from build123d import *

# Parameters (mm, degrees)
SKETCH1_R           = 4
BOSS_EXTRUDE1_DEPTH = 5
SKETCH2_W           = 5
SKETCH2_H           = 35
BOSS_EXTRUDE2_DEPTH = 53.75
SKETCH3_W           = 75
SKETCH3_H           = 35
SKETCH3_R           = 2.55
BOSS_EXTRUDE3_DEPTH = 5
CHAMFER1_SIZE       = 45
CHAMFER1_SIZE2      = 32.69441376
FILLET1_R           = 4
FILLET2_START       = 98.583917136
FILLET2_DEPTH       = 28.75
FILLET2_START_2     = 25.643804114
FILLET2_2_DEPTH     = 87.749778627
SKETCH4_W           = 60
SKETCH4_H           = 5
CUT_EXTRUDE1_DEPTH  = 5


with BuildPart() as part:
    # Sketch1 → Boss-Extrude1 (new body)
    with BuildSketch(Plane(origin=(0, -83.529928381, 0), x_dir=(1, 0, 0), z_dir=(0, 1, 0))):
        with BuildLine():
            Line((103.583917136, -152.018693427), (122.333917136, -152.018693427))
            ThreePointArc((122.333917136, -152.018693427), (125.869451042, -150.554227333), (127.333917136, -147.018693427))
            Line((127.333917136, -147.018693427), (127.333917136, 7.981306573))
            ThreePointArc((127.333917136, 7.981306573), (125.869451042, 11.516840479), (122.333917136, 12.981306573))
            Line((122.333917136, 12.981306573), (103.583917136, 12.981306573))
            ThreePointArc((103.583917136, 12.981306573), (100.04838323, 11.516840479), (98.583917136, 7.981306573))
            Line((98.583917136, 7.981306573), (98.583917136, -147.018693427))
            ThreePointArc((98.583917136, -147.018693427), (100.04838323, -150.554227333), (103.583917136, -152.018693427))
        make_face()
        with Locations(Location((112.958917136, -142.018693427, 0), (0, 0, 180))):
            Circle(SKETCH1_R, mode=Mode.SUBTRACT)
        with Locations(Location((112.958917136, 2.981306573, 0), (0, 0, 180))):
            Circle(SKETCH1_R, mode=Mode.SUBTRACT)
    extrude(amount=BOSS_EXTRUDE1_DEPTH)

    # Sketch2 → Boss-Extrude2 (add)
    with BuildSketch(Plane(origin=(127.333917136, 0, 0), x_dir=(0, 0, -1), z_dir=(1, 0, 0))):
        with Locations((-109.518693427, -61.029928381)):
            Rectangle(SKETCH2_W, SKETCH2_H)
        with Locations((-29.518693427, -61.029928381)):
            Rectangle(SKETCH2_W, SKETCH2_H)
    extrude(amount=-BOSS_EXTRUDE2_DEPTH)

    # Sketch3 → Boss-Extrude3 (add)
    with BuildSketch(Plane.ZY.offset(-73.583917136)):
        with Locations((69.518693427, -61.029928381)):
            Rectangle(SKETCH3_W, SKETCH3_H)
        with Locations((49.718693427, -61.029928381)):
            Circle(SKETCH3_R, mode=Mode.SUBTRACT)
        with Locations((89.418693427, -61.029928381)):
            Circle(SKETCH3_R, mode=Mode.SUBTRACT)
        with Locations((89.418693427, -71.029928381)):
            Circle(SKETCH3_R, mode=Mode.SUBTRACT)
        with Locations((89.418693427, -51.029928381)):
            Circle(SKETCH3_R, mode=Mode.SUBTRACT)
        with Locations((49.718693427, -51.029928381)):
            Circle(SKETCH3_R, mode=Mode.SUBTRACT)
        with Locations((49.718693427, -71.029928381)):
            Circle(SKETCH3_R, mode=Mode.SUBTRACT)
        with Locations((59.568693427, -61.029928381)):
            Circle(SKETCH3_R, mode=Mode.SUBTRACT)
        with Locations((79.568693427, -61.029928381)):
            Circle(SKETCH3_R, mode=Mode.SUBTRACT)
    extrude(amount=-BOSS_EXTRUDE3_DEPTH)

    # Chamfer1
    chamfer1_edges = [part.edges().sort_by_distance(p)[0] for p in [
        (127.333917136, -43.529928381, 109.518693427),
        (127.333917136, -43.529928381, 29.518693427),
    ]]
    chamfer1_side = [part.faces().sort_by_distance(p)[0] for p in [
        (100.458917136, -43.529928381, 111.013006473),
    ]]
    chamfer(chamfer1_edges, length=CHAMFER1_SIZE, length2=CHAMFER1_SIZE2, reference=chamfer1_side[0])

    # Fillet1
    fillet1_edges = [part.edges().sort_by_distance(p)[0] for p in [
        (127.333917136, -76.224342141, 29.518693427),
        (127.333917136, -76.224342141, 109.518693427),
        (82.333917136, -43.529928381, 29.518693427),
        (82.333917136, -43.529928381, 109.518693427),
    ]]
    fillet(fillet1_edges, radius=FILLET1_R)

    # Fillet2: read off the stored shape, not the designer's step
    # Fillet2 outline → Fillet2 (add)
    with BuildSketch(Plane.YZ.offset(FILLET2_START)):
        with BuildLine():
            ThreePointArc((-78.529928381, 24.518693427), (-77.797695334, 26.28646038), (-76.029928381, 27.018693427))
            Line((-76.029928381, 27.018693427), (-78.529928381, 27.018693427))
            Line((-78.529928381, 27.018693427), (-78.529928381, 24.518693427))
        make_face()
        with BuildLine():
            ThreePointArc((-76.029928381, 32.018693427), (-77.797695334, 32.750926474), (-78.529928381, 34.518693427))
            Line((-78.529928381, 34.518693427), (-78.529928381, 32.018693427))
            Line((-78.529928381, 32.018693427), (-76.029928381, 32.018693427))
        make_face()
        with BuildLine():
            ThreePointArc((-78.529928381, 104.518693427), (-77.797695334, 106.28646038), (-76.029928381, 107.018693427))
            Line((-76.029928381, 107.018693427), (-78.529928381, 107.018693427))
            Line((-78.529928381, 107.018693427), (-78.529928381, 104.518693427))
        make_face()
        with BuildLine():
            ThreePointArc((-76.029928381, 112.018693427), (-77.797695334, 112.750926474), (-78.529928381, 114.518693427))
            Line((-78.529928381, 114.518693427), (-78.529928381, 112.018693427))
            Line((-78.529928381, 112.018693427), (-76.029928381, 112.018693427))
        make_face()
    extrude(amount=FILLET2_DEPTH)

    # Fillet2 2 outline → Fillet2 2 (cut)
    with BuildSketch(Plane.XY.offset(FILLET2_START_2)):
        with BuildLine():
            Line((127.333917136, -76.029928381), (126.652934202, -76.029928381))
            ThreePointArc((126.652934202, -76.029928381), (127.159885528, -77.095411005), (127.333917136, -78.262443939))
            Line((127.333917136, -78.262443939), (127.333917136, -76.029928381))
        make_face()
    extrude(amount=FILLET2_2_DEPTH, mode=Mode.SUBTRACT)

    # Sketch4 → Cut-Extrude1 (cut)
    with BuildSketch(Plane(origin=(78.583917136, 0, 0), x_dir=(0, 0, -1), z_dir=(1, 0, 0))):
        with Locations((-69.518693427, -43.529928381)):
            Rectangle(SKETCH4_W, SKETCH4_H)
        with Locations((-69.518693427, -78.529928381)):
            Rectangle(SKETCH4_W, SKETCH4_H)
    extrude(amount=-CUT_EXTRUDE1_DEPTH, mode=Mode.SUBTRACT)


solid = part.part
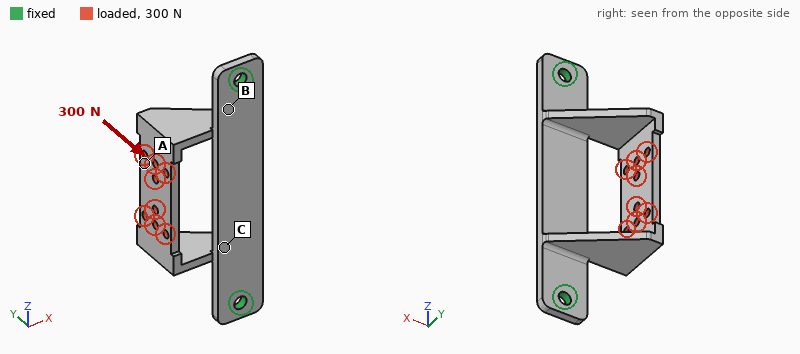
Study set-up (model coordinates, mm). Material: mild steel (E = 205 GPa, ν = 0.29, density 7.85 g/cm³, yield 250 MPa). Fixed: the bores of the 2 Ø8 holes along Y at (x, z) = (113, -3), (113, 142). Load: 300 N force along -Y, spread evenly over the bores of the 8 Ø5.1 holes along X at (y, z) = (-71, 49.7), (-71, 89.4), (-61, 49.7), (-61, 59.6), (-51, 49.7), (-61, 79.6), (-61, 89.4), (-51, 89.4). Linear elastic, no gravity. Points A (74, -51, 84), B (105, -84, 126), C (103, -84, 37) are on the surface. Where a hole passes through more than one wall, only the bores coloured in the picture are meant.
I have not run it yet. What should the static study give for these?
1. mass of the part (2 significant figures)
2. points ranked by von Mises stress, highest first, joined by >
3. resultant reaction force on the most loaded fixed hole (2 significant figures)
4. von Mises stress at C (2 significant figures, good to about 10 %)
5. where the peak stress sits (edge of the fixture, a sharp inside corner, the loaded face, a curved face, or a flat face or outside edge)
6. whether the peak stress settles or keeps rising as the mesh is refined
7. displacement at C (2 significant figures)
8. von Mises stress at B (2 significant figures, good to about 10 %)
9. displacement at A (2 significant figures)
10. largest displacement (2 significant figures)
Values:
360 g
B > C > A
160 N
9.3 MPa
edge of the fixture
keeps rising
30 µm
35 MPa
91 µm
97 µm
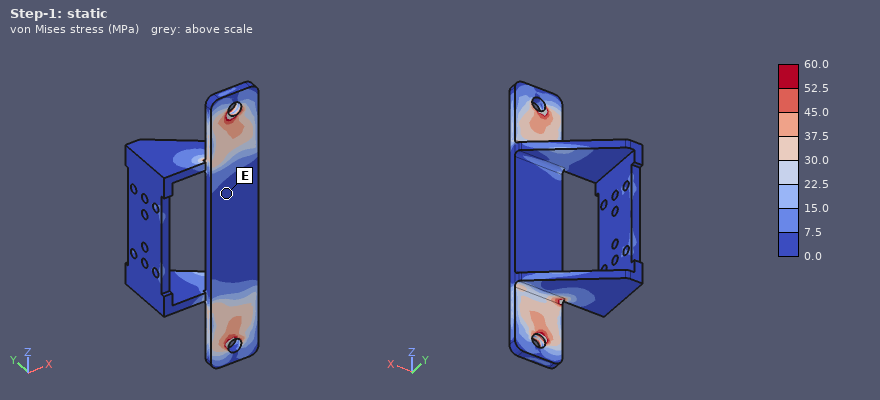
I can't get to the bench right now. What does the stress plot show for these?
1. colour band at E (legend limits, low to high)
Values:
0.0 to 7.5 MPa
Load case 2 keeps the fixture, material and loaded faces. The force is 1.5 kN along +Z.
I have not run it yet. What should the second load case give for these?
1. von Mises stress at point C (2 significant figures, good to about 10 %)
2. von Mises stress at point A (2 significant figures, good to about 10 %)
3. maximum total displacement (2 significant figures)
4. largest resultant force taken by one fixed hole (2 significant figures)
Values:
19 MPa
25 MPa
93 µm
890 N
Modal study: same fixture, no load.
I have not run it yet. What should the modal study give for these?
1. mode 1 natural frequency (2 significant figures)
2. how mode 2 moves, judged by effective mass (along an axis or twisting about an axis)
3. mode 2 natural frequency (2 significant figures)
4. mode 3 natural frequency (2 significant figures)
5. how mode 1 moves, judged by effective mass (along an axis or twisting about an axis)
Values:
780 Hz
along Y
1500 Hz
1700 Hz
along Y
